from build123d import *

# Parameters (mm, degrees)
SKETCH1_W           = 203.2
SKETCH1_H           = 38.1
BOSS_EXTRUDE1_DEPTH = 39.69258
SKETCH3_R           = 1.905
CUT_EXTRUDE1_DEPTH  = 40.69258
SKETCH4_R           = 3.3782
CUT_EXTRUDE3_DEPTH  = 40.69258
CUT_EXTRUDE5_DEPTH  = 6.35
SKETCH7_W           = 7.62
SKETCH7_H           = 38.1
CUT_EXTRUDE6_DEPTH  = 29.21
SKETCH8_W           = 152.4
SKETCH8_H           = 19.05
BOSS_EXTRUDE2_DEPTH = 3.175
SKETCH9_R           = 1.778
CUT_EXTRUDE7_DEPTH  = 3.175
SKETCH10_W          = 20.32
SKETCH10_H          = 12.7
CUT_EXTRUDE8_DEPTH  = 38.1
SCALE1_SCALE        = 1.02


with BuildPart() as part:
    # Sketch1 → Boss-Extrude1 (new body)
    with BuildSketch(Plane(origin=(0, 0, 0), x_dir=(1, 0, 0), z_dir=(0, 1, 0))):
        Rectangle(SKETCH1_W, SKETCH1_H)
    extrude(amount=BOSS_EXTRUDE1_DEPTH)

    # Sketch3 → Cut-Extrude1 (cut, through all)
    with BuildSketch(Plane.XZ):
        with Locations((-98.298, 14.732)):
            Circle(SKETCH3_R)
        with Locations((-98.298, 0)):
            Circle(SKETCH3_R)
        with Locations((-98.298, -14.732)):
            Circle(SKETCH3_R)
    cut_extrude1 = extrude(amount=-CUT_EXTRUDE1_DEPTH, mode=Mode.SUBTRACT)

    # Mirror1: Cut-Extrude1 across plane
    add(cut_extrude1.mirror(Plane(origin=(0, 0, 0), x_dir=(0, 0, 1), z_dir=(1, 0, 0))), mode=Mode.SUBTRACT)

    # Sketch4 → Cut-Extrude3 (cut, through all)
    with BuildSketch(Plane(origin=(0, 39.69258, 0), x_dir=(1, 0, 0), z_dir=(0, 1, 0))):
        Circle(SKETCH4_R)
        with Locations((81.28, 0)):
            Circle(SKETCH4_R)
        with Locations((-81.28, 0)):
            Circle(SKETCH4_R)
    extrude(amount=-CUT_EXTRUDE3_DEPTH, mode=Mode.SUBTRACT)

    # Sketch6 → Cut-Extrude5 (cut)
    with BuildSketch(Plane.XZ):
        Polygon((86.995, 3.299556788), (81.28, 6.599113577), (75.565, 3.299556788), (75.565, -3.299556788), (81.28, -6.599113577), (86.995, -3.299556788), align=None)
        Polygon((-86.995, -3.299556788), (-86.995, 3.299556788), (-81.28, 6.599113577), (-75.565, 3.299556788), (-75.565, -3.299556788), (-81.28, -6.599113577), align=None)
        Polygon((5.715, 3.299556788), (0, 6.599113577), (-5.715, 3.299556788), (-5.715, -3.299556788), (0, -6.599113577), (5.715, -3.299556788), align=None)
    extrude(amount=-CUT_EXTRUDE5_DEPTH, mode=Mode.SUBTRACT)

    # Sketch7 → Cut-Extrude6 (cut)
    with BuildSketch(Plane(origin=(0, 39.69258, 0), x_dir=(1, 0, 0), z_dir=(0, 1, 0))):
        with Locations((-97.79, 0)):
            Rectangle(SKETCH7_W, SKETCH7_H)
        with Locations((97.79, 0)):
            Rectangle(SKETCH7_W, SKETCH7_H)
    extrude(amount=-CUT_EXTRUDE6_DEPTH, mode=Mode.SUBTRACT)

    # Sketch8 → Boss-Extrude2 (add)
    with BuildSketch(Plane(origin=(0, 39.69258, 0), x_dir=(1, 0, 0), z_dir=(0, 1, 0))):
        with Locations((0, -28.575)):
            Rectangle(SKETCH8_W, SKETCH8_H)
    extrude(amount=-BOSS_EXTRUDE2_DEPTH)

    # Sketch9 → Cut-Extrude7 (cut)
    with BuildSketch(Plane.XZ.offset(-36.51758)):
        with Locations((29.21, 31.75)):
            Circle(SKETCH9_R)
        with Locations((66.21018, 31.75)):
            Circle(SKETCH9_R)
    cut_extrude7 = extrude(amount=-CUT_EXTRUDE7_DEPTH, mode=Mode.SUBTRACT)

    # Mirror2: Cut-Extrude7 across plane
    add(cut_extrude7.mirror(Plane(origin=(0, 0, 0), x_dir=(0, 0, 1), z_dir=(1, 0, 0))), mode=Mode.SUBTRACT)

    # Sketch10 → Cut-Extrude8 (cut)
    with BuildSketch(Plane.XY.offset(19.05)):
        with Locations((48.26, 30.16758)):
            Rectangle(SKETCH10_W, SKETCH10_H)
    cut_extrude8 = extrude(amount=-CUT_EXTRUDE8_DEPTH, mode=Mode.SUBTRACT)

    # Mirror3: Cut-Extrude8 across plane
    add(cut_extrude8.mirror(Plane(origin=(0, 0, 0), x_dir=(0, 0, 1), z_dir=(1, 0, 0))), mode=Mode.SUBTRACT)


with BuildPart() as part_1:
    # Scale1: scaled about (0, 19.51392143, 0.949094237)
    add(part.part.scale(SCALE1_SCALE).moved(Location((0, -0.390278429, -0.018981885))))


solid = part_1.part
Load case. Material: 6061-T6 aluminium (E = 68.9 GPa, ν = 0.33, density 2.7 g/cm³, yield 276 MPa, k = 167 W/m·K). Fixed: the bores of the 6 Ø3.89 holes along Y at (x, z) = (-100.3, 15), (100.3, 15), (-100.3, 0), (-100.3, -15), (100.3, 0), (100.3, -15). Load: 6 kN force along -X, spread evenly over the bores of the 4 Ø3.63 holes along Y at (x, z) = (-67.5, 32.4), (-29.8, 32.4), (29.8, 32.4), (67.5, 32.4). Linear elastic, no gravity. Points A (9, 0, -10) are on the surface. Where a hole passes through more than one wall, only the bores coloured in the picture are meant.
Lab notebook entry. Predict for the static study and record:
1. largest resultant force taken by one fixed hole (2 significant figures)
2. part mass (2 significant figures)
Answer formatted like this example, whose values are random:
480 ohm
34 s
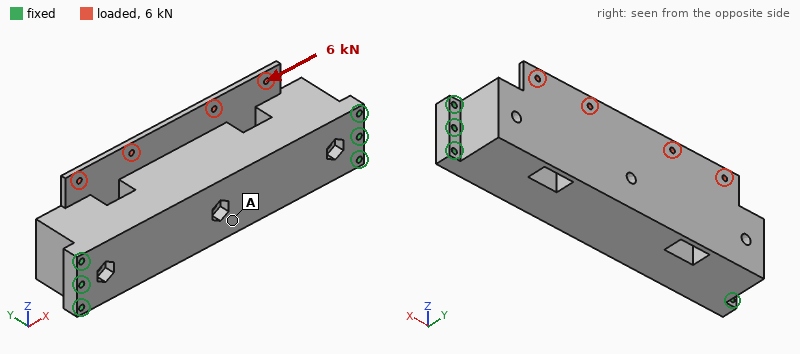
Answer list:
1.6 kN
780 g
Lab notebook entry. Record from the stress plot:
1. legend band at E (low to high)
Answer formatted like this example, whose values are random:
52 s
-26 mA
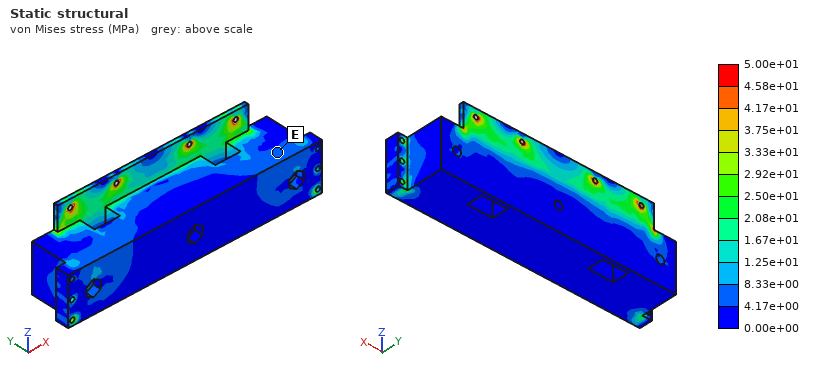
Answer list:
4.17e+00 to 8.33e+00 MPa
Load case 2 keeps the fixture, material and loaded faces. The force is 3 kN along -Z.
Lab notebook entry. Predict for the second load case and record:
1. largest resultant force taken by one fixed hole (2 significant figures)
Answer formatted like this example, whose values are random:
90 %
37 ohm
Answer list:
2.1 kN
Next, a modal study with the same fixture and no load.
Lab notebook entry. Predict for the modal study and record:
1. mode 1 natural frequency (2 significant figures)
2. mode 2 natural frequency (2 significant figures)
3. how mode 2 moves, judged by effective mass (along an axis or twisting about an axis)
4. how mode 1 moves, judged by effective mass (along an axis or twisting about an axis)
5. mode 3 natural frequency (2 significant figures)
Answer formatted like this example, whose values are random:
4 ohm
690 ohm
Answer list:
2600 Hz
2900 Hz
along Z
along Y
4100 Hz
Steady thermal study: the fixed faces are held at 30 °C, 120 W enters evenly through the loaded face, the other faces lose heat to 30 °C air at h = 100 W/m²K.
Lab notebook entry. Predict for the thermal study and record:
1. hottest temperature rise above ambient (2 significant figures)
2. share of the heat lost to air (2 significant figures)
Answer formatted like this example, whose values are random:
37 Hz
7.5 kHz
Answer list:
55 K
49 %
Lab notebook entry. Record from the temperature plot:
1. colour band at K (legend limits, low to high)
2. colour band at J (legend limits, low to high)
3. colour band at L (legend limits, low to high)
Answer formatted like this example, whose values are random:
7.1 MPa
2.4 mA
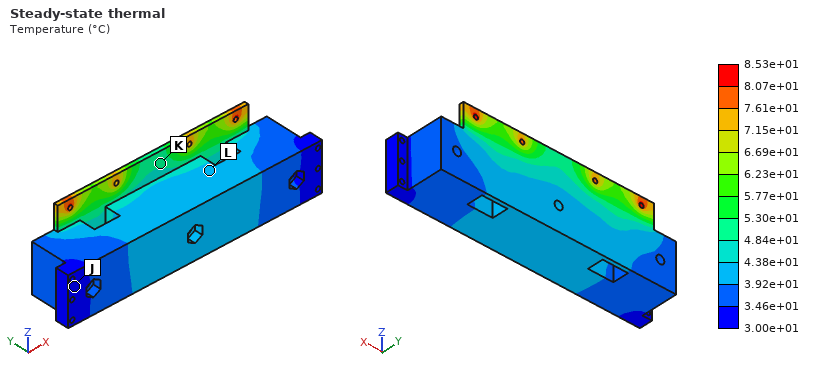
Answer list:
4.84e+01 to 5.30e+01 °C
3.00e+01 to 3.46e+01 °C
3.92e+01 to 4.38e+01 °C
